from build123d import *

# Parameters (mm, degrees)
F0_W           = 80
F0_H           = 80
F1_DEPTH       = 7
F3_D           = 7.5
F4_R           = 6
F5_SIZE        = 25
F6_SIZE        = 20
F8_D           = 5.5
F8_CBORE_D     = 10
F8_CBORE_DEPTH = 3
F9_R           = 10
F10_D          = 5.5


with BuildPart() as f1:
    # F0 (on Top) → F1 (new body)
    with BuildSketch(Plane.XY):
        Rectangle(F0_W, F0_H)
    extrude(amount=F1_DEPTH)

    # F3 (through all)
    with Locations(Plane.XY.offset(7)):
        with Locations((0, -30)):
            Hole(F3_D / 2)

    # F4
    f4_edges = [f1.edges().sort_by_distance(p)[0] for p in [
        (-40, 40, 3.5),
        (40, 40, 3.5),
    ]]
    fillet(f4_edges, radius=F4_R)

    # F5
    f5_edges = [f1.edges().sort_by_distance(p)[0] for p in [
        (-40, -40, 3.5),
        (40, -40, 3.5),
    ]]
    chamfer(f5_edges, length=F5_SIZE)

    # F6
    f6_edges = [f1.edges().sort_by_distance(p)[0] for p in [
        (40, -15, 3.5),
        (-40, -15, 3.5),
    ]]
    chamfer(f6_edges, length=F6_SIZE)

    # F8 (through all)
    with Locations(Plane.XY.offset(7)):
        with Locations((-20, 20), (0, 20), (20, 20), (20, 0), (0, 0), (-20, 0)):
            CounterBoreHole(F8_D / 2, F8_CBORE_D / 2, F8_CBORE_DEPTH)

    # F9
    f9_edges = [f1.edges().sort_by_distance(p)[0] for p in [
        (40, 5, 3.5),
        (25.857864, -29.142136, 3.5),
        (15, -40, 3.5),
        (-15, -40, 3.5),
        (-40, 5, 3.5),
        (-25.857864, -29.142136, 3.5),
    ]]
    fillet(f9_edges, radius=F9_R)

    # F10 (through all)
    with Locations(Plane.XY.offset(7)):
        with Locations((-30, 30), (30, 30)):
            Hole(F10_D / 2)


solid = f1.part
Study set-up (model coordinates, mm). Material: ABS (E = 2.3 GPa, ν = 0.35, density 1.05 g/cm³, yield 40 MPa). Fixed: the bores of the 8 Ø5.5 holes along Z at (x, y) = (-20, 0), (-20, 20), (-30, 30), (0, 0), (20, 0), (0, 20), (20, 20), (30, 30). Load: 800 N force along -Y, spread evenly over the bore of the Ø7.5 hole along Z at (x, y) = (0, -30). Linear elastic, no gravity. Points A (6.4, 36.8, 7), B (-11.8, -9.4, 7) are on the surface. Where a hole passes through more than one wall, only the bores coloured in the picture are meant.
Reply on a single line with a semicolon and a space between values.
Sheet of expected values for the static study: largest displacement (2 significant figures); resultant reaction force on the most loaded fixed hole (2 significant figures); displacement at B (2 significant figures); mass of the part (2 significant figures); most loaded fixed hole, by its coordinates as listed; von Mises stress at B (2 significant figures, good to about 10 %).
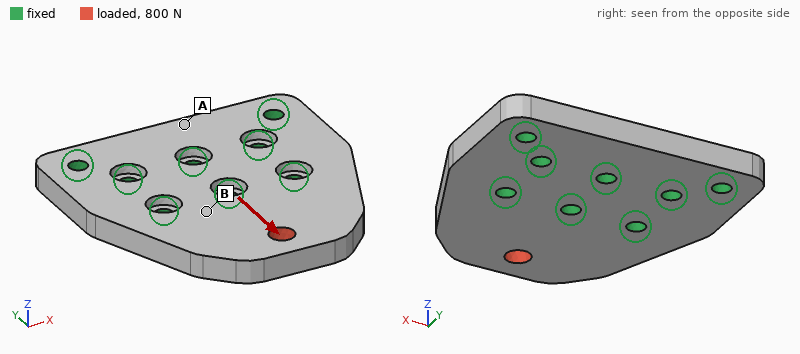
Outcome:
0.11 mm; 250 N; 0.027 mm; 37 g; (0, 0); 2.6 MPa
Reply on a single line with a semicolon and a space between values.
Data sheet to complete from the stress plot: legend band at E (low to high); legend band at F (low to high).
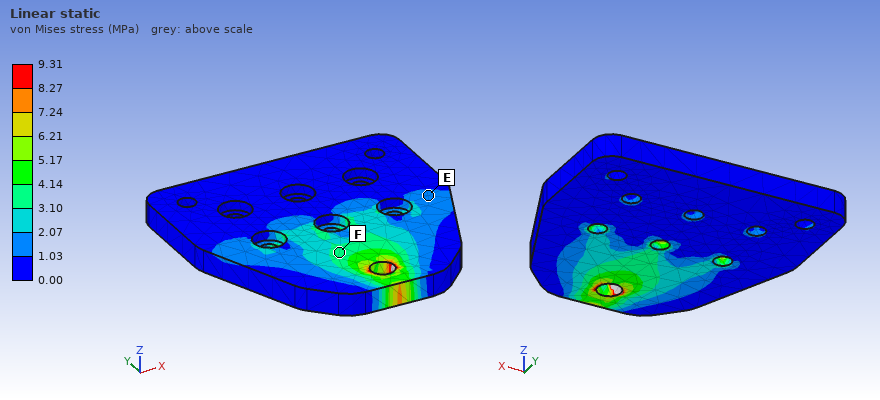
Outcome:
1.03 to 2.07 MPa; 3.10 to 4.14 MPa
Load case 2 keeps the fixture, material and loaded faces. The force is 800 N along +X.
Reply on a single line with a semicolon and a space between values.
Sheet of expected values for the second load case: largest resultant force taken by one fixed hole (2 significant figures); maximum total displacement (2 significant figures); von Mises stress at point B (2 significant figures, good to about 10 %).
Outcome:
420 N; 0.13 mm; 3.1 MPa
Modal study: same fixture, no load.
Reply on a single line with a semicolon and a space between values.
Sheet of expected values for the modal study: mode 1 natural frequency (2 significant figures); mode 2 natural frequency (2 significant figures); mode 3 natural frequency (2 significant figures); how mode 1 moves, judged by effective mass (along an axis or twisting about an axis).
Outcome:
1100 Hz; 2300 Hz; 4100 Hz; along Z
